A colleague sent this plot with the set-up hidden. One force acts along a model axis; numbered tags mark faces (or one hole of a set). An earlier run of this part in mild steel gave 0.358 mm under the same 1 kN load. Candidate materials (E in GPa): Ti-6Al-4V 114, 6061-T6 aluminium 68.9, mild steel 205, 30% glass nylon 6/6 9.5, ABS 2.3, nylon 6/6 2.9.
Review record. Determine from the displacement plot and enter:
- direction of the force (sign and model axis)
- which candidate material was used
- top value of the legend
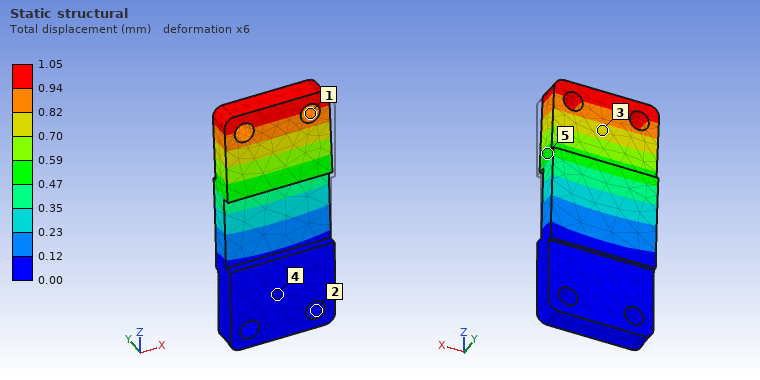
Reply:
+Y
6061-T6 aluminium
1.05 mm
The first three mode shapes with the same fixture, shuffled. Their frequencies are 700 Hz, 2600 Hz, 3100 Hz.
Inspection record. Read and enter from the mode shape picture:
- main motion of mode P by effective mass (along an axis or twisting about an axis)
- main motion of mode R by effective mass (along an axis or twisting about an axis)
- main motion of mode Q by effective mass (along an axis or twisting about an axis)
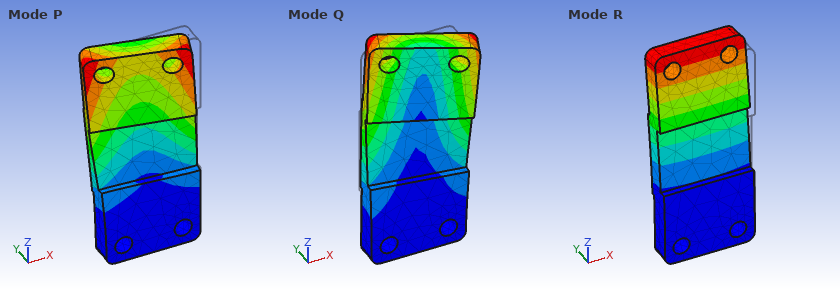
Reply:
along X
along Y
along X
